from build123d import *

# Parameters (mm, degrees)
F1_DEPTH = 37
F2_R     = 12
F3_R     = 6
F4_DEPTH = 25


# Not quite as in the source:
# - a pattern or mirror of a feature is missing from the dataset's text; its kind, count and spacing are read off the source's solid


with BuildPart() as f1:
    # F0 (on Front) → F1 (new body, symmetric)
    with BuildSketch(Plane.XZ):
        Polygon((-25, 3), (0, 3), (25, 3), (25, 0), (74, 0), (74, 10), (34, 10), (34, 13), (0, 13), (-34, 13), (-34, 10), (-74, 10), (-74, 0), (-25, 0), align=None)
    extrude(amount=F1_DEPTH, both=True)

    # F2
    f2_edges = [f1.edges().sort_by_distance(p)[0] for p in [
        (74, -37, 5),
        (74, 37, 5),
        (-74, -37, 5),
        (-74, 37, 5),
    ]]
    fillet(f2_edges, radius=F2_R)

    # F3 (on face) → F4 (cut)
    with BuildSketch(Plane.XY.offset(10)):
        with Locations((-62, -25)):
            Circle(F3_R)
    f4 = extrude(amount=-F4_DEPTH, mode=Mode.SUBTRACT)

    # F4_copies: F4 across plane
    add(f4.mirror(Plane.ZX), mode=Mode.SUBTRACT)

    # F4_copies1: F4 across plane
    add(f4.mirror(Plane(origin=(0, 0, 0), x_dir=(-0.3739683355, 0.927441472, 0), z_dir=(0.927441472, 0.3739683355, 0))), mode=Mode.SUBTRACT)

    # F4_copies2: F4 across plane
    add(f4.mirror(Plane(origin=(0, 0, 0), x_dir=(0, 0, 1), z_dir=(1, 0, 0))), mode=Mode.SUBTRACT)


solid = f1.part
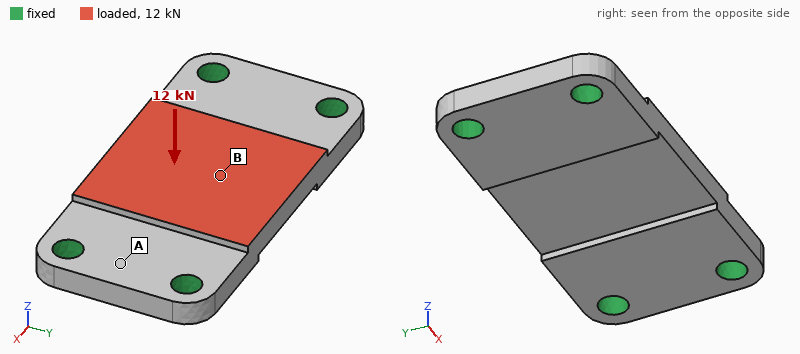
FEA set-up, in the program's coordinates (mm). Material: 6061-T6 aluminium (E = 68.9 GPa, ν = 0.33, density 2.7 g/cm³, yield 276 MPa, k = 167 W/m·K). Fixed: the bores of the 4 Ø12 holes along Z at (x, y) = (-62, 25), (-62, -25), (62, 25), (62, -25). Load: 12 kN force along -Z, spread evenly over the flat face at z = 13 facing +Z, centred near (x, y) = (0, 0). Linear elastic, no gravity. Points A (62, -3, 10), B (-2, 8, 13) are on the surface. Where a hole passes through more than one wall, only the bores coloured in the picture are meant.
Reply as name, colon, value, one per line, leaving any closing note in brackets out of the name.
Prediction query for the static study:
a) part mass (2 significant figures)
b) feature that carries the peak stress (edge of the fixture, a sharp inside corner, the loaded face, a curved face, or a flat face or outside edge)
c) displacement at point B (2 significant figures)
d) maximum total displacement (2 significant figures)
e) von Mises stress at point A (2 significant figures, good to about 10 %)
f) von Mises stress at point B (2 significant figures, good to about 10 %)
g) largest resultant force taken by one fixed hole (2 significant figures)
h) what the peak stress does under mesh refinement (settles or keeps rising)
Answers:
part mass: 290 g
feature that carries the peak stress: edge of the fixture
displacement at point B: 0.17 mm
maximum total displacement: 0.18 mm
von Mises stress at point A: 25 MPa
von Mises stress at point B: 71 MPa
largest resultant force taken by one fixed hole: 5.6 kN
what the peak stress does under mesh refinement: keeps rising
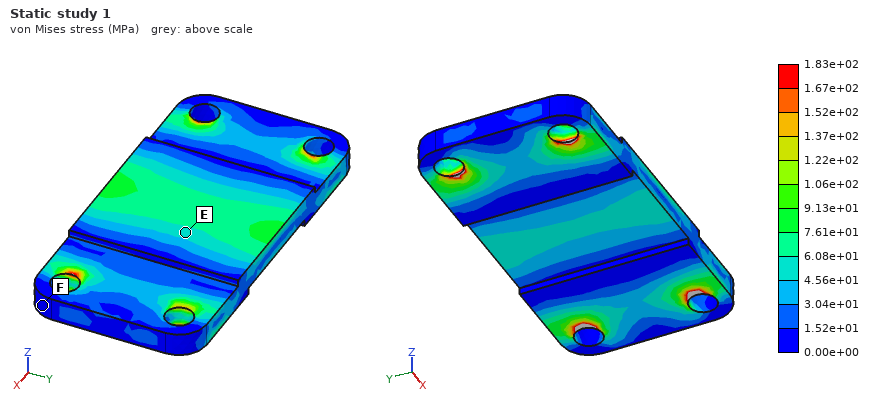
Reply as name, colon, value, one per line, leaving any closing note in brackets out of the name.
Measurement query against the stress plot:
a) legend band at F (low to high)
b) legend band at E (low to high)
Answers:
legend band at F: 0.00e+00 to 1.52e+01 MPa
legend band at E: 4.56e+01 to 6.08e+01 MPa
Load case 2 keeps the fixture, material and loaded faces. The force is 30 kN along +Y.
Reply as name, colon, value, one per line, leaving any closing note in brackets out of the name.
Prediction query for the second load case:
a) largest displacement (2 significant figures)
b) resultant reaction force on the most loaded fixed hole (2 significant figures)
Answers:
largest displacement: 0.15 mm
resultant reaction force on the most loaded fixed hole: 11 kN
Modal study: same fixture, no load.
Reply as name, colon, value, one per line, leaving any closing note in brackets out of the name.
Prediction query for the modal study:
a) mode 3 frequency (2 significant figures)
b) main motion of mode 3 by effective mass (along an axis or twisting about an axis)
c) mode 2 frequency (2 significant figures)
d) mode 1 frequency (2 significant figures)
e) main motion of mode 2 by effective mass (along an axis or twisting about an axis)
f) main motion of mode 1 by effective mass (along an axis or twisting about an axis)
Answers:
mode 3 frequency: 9000 Hz
main motion of mode 3 by effective mass: twisting about Y
mode 2 frequency: 5300 Hz
mode 1 frequency: 3700 Hz
main motion of mode 2 by effective mass: twisting about X
main motion of mode 1 by effective mass: along Z
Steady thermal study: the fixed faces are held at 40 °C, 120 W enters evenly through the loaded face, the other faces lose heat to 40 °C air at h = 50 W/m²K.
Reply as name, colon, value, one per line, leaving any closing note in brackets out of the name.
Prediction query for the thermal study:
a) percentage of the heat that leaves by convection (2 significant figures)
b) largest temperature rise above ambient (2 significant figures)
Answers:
percentage of the heat that leaves by convection: 7.8 %
largest temperature rise above ambient: 21 K
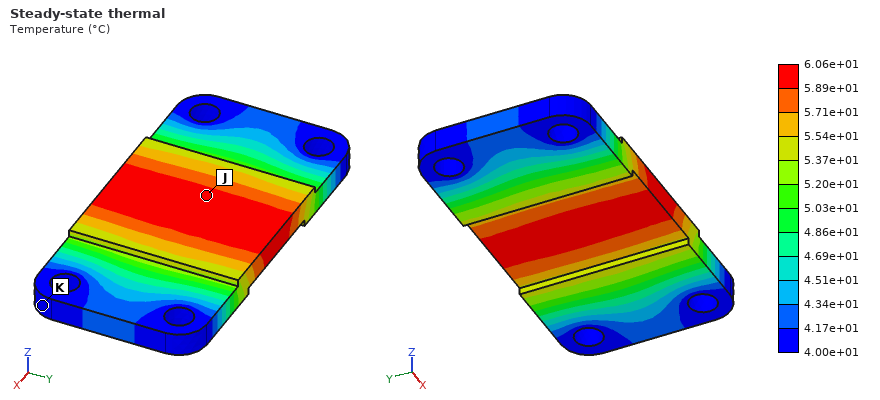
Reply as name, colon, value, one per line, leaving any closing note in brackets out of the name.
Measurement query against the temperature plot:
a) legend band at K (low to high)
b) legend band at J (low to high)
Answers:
legend band at K: 4.00e+01 to 4.17e+01 °C
legend band at J: 5.89e+01 to 6.06e+01 °C
